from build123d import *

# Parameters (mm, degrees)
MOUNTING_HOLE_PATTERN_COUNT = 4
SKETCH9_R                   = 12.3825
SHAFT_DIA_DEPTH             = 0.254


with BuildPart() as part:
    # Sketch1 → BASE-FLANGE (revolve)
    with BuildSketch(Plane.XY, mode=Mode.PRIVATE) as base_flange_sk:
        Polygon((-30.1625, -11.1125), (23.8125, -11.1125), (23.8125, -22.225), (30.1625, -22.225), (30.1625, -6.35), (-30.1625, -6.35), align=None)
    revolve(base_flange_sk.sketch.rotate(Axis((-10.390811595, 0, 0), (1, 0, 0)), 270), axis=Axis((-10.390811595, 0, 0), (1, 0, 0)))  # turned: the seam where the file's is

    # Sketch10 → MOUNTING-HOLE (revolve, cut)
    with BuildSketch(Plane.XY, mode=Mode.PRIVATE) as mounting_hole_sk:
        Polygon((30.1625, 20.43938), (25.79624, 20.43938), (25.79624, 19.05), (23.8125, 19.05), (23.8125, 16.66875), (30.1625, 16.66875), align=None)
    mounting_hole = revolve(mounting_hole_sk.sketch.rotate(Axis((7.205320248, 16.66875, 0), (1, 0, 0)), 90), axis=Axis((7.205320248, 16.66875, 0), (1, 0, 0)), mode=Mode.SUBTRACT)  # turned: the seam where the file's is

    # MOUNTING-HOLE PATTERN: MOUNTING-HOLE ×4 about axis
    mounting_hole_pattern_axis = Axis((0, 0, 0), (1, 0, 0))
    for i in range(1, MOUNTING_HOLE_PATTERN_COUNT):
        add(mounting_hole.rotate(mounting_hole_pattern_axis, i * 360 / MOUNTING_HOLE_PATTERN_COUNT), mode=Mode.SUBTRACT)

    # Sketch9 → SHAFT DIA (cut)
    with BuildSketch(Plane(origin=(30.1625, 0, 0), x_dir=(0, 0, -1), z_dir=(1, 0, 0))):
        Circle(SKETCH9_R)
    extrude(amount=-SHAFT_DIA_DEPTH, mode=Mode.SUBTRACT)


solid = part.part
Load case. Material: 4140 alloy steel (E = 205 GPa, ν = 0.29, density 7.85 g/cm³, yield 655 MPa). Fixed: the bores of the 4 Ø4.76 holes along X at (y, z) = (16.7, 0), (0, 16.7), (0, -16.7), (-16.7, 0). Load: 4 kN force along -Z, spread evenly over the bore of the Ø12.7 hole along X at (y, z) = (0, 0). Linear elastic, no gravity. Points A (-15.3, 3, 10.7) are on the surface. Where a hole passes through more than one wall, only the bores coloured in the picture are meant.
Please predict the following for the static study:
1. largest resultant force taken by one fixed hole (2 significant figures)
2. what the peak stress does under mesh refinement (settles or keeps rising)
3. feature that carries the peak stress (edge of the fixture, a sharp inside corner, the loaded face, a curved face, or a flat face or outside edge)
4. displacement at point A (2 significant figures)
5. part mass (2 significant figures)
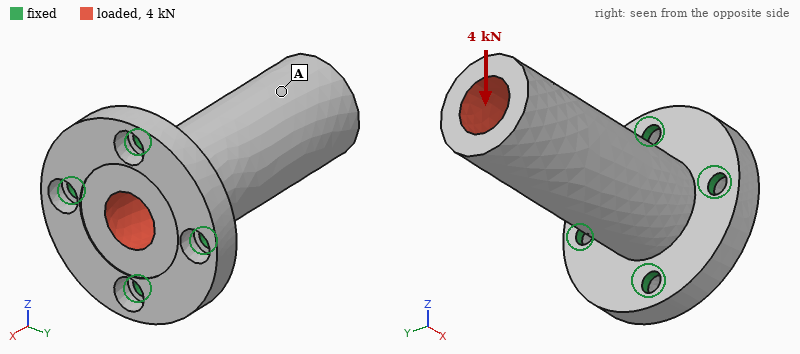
3.1 kN
keeps rising
edge of the fixture
64 µm
170 g
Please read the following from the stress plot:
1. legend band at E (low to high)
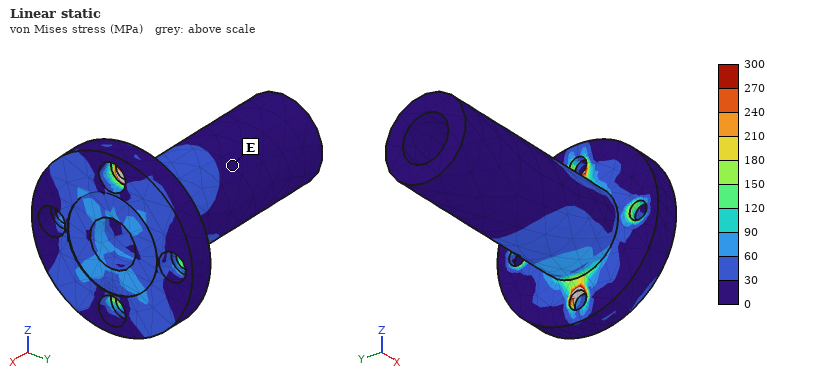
0 to 30 MPa
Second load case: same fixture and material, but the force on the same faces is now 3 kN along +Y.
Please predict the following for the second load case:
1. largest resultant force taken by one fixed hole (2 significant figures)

2.4 kN
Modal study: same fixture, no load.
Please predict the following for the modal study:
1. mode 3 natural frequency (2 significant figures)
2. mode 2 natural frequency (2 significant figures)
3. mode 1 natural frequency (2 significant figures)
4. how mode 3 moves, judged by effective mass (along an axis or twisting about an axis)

13 kHz
3700 Hz
3700 Hz
along X
